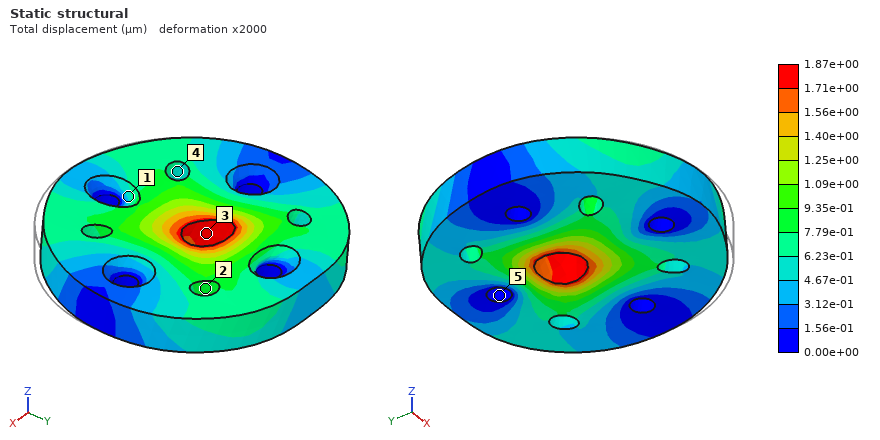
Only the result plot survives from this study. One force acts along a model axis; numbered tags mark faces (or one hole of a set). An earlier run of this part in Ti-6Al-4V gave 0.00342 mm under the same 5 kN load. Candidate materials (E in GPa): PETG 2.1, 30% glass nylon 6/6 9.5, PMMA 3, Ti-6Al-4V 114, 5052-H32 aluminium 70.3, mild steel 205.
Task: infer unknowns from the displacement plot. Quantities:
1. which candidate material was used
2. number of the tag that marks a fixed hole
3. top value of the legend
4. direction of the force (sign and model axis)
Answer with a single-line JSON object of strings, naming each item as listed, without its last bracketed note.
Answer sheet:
{"which candidate material was used": "mild steel", "number of the tag that marks a fixed hole": "5", "top value of the legend": "1.87e+00 µm", "direction of the force": "+Y"}
